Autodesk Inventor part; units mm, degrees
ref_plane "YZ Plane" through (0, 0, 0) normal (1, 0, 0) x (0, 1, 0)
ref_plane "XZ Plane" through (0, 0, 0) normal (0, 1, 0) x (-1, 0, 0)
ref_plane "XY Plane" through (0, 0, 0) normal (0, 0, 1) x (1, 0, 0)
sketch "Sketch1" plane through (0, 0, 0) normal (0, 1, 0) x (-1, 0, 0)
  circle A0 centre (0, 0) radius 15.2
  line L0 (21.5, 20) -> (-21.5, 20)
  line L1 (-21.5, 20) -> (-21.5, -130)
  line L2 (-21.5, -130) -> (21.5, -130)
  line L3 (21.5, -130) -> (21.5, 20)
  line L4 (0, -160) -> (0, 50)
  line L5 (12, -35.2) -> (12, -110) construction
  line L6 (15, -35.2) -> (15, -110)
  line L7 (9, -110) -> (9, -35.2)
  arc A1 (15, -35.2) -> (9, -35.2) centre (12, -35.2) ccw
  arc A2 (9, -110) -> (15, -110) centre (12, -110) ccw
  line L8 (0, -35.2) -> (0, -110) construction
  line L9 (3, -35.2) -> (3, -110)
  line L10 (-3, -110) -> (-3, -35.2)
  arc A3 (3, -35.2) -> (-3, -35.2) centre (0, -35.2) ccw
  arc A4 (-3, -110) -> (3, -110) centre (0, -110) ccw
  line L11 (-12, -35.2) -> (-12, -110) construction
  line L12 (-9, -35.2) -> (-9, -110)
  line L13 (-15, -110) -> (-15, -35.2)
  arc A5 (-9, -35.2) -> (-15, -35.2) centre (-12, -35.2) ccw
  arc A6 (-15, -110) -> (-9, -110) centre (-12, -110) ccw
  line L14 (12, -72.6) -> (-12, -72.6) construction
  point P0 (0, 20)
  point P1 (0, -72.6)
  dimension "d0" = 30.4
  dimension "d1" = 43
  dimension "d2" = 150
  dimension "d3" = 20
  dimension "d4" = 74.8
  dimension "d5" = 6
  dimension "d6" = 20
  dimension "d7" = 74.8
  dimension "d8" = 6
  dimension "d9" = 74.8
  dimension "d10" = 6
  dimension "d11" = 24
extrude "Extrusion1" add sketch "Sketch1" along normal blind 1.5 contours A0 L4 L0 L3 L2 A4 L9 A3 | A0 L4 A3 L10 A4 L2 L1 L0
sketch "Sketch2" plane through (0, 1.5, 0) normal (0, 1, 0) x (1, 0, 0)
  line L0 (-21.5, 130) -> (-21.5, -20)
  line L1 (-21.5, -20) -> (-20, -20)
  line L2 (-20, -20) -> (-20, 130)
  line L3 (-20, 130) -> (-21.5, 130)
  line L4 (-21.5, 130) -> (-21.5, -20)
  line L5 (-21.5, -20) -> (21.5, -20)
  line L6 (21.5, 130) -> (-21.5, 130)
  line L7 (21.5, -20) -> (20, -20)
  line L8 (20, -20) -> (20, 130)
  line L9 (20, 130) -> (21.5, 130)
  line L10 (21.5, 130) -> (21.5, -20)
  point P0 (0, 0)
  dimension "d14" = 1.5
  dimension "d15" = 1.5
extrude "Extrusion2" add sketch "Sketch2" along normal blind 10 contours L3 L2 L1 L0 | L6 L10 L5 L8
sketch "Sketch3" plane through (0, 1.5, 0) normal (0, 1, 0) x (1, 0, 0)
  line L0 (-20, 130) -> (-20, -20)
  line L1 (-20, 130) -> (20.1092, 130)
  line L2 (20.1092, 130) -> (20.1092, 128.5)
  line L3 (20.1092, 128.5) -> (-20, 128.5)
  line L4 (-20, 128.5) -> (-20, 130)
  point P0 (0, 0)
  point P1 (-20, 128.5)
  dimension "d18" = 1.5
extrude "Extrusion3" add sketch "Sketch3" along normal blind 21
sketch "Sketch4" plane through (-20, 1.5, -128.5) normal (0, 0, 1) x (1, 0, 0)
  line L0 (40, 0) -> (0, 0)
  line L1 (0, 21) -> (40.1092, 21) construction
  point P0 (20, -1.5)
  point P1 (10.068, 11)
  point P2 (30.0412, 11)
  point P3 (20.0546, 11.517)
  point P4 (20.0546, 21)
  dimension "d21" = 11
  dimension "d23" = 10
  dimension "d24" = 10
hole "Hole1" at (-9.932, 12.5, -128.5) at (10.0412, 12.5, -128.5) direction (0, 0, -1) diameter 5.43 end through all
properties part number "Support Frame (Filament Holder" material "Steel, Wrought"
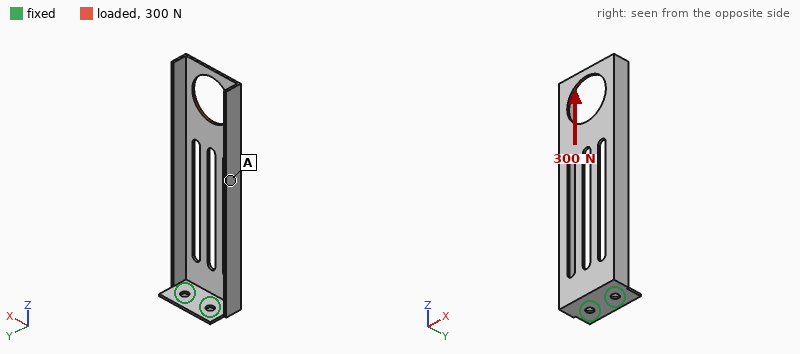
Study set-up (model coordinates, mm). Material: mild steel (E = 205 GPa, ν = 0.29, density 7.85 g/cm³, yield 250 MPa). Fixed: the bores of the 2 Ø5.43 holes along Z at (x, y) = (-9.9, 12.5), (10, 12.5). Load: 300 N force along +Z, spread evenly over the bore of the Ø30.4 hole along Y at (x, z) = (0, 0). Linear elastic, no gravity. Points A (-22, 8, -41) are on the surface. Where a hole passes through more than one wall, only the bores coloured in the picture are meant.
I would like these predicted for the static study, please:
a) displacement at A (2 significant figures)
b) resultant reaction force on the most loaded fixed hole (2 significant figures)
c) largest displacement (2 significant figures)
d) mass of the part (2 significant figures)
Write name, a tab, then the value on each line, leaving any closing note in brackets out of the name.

displacement at A	0.39 mm
resultant reaction force on the most loaded fixed hole	150 N
largest displacement	0.68 mm
mass of the part	95 g
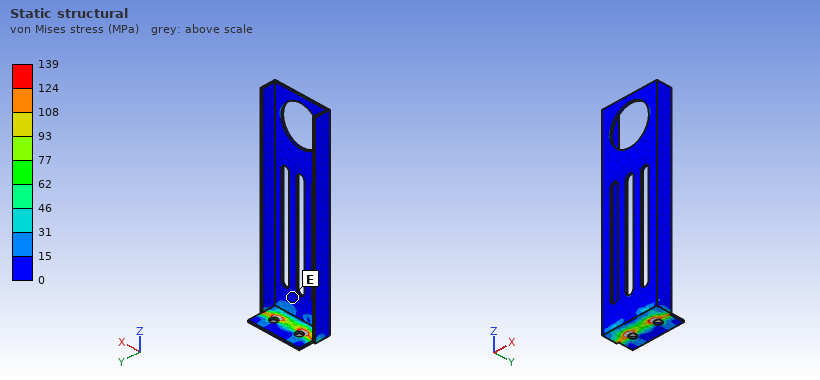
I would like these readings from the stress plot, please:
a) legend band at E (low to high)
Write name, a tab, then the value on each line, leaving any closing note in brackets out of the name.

legend band at E	0 to 15 MPa
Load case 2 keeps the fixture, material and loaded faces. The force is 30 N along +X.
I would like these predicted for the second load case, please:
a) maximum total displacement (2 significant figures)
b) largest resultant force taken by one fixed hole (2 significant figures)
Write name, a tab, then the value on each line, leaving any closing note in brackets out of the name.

maximum total displacement	0.34 mm
largest resultant force taken by one fixed hole	140 N
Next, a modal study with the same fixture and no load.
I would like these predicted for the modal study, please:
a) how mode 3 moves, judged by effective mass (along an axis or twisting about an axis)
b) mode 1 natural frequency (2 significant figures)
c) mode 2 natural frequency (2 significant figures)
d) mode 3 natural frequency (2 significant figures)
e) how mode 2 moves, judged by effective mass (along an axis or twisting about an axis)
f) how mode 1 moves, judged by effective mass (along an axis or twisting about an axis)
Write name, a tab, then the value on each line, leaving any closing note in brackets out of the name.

how mode 3 moves, judged by effective mass	along X
mode 1 natural frequency	130 Hz
mode 2 natural frequency	240 Hz
mode 3 natural frequency	480 Hz
how mode 2 moves, judged by effective mass	along X
how mode 1 moves, judged by effective mass	along Y
